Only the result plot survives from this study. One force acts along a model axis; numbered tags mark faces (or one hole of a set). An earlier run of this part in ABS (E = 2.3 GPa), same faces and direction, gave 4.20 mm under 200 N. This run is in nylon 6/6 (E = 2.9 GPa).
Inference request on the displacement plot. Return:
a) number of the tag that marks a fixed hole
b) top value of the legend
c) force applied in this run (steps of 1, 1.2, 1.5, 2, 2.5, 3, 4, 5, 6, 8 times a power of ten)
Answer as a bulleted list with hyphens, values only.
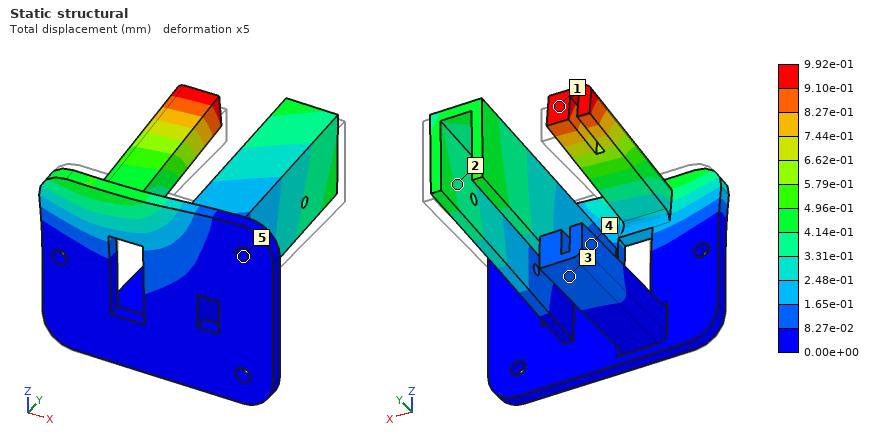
- 5
- 9.92e-01 mm
- 60 N
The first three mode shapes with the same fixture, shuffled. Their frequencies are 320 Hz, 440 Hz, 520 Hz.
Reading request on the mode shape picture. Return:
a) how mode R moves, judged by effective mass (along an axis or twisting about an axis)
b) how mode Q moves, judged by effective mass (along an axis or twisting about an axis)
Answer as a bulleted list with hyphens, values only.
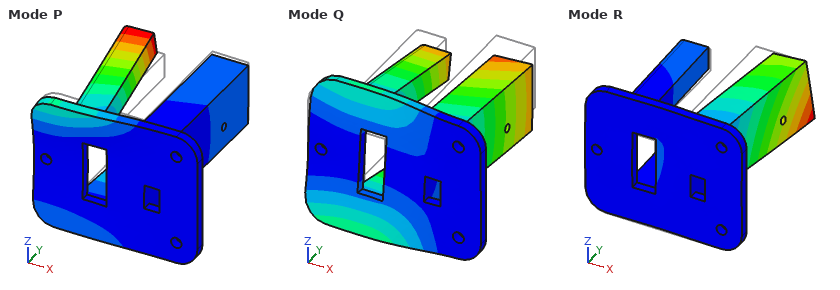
- along X
- along Z
